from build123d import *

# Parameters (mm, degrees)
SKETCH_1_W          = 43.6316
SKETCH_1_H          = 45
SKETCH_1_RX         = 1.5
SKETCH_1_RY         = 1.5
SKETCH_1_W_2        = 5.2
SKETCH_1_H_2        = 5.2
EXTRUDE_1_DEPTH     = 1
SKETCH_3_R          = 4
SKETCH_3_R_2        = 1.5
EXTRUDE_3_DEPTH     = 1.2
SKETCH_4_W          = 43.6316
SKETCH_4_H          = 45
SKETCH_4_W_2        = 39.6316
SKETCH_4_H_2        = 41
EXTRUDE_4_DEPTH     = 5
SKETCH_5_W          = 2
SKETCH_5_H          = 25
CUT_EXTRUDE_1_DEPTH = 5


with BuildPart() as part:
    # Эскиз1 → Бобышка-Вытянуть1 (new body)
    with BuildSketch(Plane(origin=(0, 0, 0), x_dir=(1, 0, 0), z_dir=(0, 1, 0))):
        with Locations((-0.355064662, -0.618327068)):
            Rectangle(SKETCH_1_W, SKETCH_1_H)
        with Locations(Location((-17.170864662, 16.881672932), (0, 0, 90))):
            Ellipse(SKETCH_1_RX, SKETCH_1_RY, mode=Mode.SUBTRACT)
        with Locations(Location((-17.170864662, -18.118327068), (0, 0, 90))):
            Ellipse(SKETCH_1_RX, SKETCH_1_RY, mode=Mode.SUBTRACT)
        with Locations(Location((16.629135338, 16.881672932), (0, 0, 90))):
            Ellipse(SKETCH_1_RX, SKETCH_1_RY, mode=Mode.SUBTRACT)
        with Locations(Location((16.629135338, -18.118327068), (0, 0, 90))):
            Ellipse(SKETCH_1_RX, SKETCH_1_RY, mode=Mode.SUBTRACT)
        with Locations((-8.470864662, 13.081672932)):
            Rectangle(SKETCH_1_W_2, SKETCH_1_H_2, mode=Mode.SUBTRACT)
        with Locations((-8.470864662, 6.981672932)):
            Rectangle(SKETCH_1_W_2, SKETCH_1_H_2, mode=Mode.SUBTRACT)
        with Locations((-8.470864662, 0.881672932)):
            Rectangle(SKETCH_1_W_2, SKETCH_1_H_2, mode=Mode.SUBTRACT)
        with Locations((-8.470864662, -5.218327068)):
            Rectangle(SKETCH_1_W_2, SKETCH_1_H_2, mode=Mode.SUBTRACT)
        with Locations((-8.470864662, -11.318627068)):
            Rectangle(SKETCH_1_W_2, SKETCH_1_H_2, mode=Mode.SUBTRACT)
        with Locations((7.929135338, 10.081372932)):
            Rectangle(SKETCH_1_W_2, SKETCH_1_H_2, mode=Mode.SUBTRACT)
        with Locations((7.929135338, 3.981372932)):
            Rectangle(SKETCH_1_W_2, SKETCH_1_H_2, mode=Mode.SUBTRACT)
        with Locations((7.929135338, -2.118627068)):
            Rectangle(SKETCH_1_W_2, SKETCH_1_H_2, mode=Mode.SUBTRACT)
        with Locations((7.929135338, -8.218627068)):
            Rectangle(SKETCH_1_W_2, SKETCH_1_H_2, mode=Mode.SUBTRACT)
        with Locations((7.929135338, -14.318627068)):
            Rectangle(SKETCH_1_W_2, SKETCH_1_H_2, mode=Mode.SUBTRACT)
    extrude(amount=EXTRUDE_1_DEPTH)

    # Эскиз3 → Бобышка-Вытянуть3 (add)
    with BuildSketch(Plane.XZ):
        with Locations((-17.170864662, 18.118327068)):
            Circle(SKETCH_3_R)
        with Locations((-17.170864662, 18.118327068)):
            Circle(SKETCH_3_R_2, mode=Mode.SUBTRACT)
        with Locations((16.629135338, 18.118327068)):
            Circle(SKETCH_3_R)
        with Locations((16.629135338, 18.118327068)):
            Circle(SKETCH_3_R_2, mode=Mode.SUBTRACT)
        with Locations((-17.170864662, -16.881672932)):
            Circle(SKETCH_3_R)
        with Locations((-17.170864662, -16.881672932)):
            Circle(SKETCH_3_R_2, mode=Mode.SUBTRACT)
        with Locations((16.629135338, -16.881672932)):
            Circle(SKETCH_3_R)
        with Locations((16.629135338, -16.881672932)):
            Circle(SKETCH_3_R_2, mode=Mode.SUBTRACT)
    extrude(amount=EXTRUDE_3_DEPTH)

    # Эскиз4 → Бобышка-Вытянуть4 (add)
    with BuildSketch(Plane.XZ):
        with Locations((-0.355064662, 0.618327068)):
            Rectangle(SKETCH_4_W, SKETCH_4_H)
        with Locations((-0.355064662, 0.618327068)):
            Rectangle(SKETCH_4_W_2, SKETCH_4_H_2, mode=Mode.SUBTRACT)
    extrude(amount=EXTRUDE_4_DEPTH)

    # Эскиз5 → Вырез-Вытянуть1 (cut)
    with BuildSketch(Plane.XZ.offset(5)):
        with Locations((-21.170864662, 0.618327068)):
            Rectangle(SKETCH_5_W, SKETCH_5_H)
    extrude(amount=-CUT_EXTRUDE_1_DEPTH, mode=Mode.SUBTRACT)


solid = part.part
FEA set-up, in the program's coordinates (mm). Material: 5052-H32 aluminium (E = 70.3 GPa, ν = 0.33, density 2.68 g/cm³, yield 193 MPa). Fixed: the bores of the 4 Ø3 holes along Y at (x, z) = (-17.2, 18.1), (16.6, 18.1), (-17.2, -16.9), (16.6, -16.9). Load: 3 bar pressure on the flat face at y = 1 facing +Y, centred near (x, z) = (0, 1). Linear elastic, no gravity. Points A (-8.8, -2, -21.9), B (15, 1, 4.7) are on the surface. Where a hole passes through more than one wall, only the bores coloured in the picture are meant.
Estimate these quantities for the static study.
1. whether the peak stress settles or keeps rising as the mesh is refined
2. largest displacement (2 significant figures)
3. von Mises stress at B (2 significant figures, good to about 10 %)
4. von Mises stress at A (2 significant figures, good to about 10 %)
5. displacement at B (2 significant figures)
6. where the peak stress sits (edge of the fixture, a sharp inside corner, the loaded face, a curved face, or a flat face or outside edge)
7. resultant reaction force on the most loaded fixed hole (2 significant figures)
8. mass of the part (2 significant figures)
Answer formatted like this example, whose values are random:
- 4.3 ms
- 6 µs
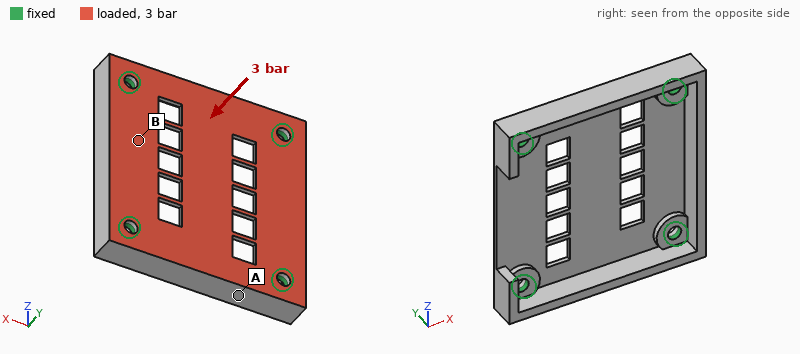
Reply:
- keeps rising
- 0.21 mm
- 43 MPa
- 16 MPa
- 0.047 mm
- edge of the fixture
- 160 N
- 8.8 g
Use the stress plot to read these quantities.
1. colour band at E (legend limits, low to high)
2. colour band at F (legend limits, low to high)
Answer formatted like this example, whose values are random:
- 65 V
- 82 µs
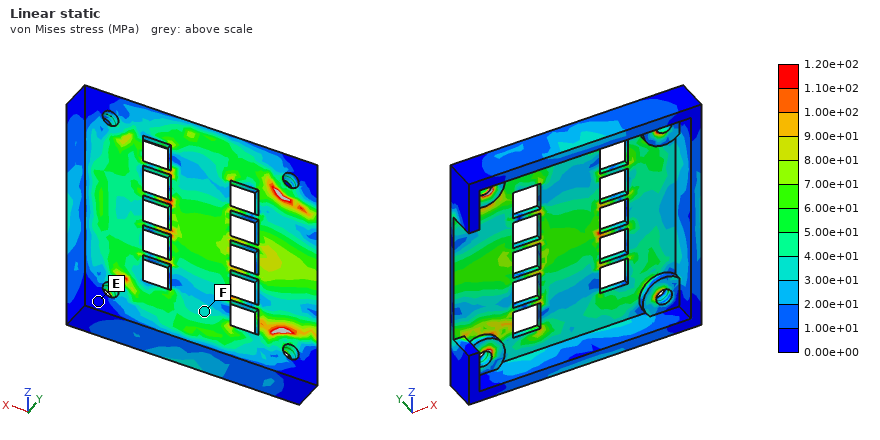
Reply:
- 0.00e+00 to 1.00e+01 MPa
- 3.00e+01 to 4.00e+01 MPa
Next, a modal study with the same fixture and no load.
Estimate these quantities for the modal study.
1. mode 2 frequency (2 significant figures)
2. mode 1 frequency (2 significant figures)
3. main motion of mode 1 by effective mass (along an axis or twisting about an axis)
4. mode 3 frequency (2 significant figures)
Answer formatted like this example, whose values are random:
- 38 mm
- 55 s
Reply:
- 7300 Hz
- 4600 Hz
- along Y
- 9300 Hz
